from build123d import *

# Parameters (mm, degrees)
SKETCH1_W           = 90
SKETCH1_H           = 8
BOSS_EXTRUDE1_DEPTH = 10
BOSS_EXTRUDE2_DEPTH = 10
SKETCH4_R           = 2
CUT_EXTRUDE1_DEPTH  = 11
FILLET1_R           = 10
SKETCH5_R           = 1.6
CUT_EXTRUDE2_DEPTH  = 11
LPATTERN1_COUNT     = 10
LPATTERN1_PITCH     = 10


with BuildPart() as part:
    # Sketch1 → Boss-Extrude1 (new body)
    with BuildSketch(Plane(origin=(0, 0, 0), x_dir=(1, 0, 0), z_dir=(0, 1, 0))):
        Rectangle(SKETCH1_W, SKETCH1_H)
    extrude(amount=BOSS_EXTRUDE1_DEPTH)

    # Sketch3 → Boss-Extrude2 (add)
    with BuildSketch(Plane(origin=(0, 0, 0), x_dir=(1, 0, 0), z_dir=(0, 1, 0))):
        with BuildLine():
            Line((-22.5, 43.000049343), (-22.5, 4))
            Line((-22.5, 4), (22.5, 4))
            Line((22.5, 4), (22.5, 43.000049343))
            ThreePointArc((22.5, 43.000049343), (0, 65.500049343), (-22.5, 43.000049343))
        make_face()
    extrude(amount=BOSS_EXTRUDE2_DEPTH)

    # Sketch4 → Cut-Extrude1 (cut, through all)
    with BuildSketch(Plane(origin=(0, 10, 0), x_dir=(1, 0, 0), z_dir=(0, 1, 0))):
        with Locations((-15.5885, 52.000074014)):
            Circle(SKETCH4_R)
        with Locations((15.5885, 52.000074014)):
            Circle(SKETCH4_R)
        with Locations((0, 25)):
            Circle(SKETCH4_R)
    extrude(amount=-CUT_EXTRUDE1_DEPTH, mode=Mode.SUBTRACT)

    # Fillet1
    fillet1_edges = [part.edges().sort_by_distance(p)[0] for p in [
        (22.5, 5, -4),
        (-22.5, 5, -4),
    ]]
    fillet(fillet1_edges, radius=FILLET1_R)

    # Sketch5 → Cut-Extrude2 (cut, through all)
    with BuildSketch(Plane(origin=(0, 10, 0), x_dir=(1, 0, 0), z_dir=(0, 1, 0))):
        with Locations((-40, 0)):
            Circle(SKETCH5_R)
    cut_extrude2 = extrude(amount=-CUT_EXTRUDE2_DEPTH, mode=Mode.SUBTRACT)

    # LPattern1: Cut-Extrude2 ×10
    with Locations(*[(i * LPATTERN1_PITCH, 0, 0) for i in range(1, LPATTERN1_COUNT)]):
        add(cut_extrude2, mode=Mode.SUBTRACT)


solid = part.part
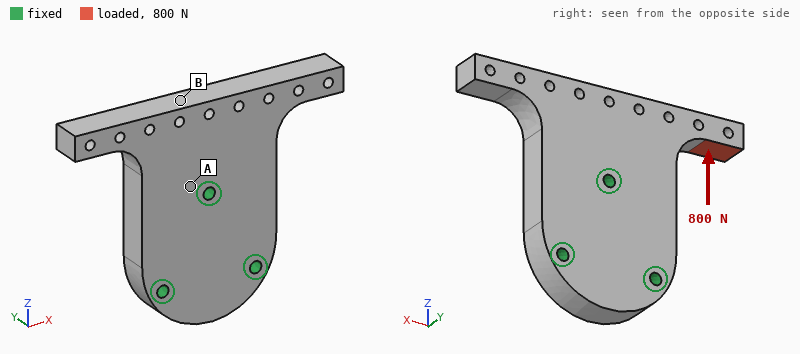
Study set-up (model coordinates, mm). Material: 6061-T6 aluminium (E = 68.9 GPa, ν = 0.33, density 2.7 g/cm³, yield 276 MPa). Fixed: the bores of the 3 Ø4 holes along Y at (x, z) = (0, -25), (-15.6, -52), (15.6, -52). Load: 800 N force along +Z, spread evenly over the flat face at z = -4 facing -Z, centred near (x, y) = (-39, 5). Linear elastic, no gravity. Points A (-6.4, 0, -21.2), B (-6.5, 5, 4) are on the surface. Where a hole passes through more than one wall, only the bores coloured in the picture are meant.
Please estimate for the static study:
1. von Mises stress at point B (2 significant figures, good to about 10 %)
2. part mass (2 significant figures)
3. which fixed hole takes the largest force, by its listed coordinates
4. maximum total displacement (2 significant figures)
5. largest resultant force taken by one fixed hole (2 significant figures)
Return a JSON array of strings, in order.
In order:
["16 MPa", "86 g", "(-15.6, -52)", "91 µm", "760 N"]
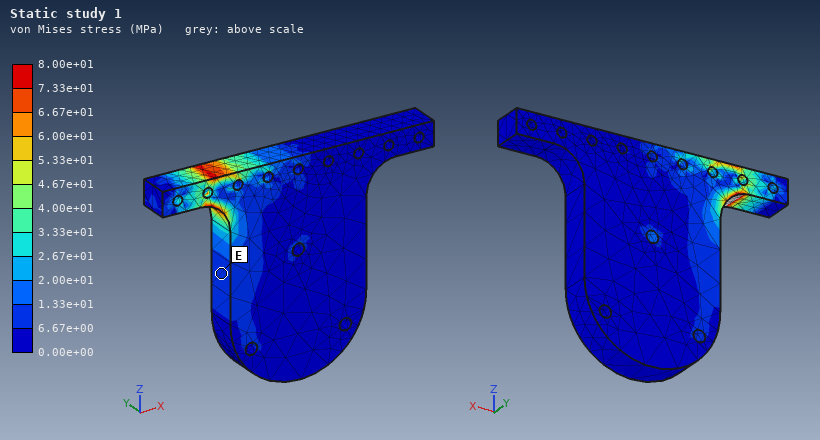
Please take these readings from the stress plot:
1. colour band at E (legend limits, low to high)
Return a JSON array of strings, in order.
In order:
["6.67e+00 to 1.33e+01 MPa"]
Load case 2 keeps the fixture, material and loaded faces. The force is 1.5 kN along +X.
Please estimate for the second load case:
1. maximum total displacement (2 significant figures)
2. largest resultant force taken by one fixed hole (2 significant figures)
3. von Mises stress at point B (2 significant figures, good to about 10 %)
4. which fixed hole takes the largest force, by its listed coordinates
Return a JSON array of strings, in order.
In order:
["32 µm", "1.9 kN", "9.8 MPa", "(0, -25)"]
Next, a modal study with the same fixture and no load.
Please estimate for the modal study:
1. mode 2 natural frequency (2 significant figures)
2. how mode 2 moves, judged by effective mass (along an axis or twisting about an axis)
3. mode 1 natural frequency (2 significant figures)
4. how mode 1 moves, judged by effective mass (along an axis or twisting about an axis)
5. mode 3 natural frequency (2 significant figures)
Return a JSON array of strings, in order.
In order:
["4900 Hz", "along Y", "4300 Hz", "twisting about Z", "8600 Hz"]
